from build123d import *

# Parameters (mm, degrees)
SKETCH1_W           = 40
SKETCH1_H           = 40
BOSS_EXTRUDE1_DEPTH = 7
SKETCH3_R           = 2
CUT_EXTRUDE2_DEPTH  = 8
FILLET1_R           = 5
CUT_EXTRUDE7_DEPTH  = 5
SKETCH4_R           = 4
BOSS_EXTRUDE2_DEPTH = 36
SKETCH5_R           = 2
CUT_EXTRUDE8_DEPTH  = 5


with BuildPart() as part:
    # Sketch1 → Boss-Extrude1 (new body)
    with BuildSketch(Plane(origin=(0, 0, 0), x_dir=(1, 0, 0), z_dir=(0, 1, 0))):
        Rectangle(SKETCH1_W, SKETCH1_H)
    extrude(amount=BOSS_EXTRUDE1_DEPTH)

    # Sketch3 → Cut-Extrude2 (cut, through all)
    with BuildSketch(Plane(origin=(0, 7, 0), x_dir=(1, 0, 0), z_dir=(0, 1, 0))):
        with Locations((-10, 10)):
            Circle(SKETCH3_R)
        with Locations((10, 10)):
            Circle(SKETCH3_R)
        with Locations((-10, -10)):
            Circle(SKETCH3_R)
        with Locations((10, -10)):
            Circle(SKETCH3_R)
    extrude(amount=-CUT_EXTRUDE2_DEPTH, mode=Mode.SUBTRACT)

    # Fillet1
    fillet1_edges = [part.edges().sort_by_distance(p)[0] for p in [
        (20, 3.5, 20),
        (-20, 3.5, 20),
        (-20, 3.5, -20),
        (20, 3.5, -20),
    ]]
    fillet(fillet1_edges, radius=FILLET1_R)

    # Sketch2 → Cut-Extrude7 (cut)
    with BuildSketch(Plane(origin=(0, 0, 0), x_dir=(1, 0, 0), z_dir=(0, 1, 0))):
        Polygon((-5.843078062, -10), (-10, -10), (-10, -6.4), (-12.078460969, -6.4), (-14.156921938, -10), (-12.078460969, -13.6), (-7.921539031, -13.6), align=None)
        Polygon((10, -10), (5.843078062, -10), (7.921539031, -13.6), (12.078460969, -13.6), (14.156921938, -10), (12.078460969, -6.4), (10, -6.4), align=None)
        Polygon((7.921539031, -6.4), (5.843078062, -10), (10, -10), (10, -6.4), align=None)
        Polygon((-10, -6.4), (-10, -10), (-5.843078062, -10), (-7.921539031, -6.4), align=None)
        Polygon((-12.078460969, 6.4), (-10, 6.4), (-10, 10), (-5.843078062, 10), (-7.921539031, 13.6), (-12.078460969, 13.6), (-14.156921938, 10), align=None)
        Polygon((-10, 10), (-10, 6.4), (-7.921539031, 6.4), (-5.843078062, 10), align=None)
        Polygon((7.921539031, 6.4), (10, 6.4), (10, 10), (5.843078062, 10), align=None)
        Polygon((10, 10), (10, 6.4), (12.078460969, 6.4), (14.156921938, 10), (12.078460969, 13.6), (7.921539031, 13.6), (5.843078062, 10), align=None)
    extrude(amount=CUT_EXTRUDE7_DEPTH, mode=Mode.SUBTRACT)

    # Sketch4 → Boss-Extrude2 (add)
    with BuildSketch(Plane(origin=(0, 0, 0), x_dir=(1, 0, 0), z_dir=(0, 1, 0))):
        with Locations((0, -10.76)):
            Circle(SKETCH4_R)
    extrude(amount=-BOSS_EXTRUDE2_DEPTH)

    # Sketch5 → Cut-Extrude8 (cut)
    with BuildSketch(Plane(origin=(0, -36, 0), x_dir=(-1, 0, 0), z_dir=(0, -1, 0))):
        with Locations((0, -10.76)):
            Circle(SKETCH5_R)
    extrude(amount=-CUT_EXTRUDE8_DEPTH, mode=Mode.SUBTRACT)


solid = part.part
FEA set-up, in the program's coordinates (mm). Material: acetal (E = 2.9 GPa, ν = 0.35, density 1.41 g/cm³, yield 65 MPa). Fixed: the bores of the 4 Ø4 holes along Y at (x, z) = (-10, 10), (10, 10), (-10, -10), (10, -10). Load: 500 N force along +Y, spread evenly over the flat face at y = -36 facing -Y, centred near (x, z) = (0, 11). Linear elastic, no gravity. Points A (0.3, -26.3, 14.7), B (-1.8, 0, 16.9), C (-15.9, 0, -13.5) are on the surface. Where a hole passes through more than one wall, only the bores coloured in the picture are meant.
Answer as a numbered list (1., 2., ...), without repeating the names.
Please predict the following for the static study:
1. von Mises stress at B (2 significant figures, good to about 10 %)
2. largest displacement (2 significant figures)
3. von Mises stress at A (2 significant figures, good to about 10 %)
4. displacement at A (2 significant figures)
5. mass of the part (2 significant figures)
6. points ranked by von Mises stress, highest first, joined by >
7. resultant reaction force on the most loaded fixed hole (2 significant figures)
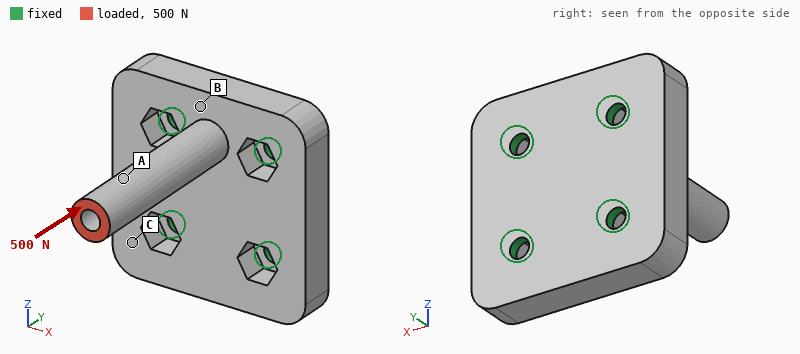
1. 6.4 MPa
2. 0.25 mm
3. 10 MPa
4. 0.19 mm
5. 17 g
6. A > B > C
7. 270 N
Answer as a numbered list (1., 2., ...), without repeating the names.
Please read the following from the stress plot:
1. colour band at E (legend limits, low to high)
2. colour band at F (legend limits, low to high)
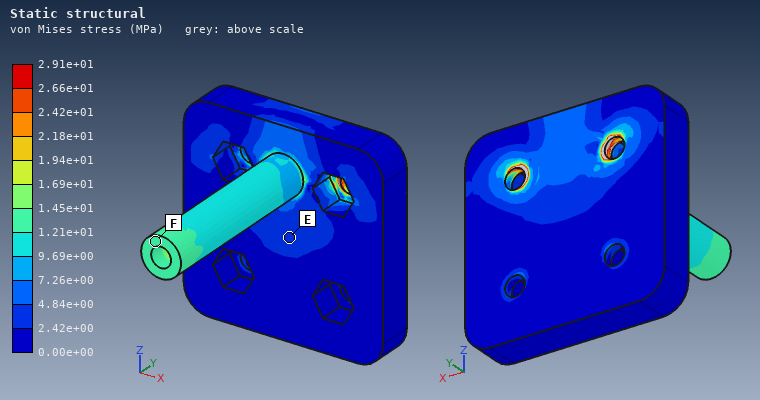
1. 2.42e+00 to 4.84e+00 MPa
2. 1.21e+01 to 1.45e+01 MPa
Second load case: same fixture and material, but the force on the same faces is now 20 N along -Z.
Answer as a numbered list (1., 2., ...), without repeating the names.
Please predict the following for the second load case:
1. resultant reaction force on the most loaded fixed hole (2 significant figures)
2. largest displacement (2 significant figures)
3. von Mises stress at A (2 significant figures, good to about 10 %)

1. 30 N
2. 0.71 mm
3. 3.8 MPa
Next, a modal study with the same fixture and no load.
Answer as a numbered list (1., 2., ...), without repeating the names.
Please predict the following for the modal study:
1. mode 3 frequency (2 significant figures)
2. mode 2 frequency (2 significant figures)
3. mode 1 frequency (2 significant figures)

1. 5000 Hz
2. 1100 Hz
3. 1100 Hz
